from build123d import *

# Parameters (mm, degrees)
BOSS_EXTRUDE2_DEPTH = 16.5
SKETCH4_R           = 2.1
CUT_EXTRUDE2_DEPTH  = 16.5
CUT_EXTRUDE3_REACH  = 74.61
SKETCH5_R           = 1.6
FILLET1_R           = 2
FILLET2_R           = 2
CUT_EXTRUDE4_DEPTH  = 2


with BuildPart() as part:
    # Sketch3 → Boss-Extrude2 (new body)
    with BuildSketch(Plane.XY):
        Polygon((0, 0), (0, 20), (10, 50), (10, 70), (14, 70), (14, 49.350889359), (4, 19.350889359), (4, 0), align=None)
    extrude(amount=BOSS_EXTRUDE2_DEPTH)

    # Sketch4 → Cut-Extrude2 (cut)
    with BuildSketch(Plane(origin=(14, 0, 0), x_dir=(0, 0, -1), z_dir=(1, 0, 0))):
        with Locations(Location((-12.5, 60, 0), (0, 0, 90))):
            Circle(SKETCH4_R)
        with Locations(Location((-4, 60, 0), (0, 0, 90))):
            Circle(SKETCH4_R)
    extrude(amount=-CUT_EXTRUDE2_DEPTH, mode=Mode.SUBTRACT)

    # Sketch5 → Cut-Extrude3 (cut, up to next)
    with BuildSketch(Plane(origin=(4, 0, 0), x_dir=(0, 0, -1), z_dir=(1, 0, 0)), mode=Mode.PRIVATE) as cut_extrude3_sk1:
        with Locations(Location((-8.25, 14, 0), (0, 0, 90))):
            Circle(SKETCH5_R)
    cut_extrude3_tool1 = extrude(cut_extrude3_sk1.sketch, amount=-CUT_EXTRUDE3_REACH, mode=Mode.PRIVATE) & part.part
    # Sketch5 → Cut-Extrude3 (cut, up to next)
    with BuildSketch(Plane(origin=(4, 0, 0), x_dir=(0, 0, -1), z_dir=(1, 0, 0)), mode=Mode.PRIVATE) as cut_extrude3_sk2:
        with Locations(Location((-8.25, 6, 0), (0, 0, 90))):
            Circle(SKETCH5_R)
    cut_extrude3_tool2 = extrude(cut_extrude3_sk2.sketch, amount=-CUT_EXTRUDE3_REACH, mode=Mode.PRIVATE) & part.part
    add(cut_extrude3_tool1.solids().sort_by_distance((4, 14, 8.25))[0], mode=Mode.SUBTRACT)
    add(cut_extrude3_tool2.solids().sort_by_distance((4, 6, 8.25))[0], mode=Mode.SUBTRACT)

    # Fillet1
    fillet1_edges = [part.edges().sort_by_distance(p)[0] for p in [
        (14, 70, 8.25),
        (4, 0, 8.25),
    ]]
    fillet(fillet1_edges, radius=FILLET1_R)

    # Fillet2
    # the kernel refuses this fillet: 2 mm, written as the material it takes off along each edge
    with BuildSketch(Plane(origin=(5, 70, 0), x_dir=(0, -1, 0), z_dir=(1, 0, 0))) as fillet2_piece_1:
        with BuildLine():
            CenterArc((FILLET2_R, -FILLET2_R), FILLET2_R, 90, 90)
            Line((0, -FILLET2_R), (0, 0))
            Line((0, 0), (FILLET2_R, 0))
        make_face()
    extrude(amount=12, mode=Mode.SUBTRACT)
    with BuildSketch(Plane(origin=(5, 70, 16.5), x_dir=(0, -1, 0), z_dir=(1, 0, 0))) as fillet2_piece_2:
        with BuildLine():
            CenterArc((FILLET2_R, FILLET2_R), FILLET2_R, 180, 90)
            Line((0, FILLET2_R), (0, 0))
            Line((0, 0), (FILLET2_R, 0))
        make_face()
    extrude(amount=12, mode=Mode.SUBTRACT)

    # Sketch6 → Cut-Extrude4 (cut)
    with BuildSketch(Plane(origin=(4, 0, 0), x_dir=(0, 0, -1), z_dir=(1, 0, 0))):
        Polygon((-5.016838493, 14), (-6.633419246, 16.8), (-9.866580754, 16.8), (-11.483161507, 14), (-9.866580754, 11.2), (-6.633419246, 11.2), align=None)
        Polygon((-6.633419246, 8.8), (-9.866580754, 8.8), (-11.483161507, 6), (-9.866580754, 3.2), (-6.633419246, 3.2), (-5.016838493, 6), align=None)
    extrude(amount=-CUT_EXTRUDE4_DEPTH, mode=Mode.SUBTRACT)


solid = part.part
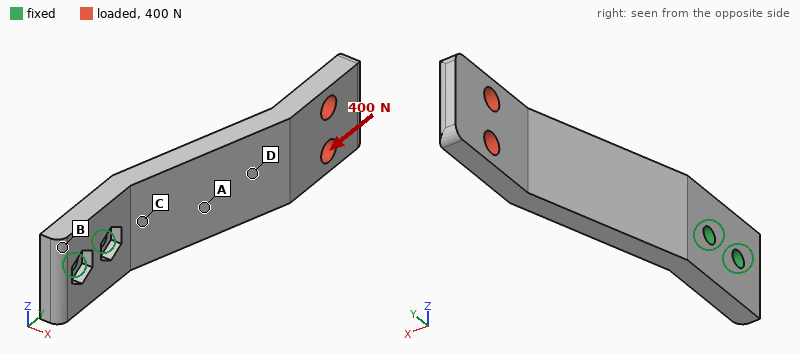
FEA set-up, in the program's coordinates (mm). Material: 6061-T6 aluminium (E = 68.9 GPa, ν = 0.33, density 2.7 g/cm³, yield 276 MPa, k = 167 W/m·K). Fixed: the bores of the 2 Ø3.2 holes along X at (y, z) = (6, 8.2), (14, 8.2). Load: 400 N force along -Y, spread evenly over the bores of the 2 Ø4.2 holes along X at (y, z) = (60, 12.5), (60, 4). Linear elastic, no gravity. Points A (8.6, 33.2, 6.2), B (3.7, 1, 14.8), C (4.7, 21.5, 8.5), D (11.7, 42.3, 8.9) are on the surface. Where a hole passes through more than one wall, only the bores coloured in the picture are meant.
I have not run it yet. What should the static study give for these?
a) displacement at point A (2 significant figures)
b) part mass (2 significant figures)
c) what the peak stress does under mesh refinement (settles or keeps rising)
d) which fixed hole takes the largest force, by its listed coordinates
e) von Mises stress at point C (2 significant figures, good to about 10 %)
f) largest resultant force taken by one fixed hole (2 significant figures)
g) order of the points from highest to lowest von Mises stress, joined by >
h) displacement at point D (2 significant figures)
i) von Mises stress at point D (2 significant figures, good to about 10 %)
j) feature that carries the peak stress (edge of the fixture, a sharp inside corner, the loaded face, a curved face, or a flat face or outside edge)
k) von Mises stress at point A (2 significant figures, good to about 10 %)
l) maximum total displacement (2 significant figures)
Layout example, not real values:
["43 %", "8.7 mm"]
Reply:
["0.18 mm", "12 g", "keeps rising", "(6, 8.2)", "74 MPa", "560 N", "C > A > D > B", "0.32 mm", "26 MPa", "edge of the fixture", "53 MPa", "0.76 mm"]
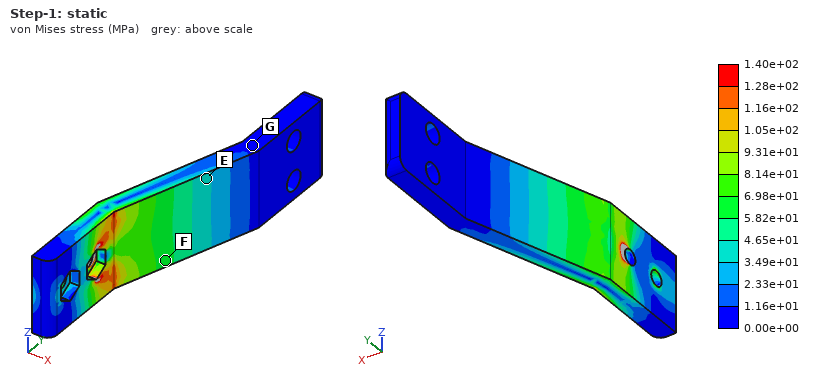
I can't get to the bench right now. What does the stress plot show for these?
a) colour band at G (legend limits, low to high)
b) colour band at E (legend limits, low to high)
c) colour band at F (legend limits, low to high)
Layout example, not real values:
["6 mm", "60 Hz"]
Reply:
["0.00e+00 to 1.16e+01 MPa", "3.49e+01 to 4.65e+01 MPa", "5.82e+01 to 6.98e+01 MPa"]
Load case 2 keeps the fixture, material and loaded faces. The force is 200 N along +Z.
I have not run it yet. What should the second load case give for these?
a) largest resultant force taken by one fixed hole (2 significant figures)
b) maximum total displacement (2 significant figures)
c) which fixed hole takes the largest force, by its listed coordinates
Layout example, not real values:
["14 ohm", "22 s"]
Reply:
["950 N", "0.20 mm", "(14, 8.2)"]
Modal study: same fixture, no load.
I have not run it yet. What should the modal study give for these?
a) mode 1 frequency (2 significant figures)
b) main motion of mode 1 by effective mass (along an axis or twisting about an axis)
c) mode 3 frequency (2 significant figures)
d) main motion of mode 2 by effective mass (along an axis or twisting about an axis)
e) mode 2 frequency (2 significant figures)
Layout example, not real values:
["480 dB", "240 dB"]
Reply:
["940 Hz", "along X", "5300 Hz", "along Z", "2700 Hz"]
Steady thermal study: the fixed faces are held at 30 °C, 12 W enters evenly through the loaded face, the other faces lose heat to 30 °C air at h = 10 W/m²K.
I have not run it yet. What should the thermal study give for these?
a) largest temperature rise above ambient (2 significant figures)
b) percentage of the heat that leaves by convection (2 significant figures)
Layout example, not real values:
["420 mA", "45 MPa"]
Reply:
["55 K", "6.4 %"]
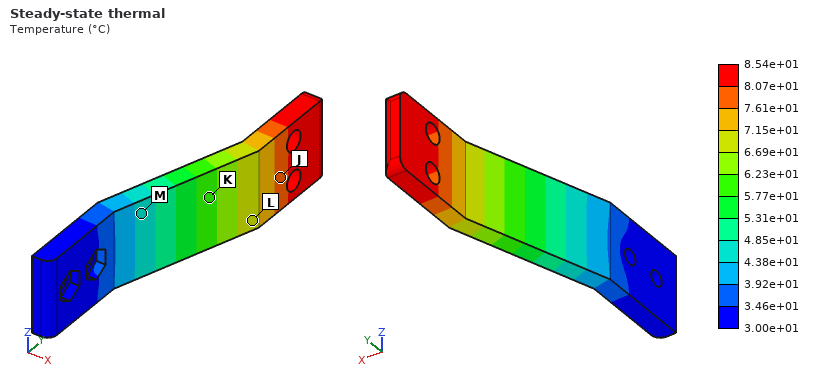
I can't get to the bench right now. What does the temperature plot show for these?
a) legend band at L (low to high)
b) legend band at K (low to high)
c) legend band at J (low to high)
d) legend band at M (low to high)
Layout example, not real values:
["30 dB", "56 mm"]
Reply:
["6.69e+01 to 7.15e+01 °C", "5.77e+01 to 6.23e+01 °C", "7.61e+01 to 8.07e+01 °C", "4.38e+01 to 4.85e+01 °C"]
